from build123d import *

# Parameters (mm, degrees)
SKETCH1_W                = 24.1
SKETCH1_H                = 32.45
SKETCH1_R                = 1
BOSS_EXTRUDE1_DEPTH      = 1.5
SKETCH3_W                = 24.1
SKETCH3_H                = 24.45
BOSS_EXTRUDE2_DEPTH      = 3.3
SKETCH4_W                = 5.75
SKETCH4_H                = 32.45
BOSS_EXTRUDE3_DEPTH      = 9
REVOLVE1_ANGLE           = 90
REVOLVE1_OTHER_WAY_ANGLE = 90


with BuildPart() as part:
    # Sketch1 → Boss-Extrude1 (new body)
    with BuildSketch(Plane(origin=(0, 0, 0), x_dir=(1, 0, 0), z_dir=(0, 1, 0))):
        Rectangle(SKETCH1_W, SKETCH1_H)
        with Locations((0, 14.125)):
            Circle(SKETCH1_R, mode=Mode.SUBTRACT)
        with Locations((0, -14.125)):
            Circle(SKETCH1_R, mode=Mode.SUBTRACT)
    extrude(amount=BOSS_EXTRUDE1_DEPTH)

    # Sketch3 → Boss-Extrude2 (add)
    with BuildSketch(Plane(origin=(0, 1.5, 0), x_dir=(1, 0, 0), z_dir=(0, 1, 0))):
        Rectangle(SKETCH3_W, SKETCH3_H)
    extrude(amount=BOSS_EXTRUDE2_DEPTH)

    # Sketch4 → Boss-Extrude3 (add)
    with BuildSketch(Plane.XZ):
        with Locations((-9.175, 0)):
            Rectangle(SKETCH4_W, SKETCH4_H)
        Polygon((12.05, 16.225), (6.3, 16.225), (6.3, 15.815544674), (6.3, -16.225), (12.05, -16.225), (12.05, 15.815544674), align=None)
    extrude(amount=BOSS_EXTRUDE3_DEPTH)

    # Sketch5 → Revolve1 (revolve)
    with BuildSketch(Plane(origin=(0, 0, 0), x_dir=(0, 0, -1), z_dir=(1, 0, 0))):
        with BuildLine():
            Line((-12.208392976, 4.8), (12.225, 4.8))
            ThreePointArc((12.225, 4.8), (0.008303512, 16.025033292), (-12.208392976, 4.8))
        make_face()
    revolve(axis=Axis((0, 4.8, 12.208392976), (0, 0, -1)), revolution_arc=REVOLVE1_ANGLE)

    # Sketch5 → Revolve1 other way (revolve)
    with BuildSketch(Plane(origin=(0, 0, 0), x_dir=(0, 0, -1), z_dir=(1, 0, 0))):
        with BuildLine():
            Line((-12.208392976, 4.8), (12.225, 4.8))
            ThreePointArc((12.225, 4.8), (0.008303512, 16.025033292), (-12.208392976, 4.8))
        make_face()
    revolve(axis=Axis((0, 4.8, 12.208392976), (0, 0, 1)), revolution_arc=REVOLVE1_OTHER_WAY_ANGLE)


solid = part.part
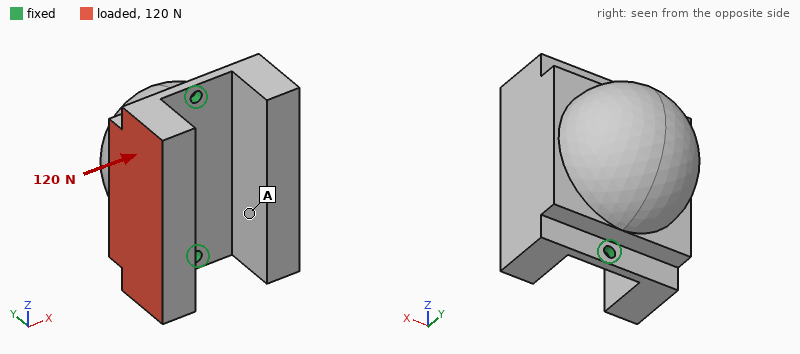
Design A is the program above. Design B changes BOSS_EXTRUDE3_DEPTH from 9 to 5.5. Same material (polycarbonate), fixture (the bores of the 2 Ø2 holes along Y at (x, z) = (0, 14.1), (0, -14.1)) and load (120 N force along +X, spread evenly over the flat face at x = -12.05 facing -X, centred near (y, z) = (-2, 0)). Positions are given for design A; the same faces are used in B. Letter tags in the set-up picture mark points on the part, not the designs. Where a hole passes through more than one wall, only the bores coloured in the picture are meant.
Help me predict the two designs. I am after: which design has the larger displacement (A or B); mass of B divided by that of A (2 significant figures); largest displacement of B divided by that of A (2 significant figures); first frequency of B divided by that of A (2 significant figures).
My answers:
A
0.86
0.40
1.1
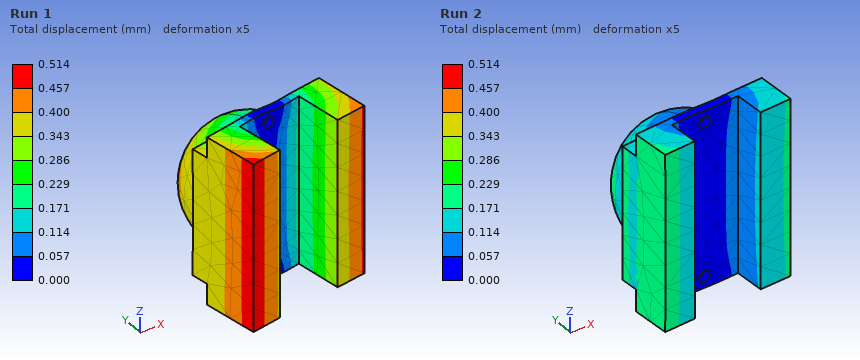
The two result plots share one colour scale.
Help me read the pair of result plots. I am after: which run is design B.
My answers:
Run 2
